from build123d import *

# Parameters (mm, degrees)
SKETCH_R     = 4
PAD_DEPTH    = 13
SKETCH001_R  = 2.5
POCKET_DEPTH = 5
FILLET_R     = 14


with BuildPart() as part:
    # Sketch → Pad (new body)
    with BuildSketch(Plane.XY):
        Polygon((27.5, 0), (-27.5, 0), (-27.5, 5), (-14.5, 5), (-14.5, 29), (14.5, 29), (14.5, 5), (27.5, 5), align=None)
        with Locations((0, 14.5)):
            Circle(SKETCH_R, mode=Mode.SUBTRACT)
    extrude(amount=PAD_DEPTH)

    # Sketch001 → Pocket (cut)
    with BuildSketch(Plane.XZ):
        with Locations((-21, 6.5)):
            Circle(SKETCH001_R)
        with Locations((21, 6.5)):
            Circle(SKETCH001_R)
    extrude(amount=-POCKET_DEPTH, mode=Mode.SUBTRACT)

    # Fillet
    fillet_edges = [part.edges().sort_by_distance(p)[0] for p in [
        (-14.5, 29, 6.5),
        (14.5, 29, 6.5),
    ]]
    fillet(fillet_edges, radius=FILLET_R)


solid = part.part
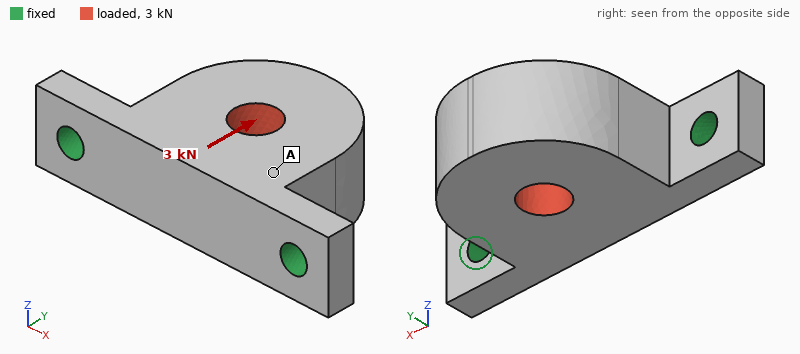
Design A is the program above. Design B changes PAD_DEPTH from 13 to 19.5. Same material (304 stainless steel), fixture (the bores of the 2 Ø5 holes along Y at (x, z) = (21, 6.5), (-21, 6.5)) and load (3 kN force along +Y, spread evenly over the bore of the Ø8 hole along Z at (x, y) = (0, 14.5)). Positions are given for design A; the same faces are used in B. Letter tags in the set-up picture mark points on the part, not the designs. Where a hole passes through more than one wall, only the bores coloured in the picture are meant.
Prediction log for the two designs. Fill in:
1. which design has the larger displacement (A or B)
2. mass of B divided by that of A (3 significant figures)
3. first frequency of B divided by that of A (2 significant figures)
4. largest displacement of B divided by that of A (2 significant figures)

B
1.51
0.94
2.5
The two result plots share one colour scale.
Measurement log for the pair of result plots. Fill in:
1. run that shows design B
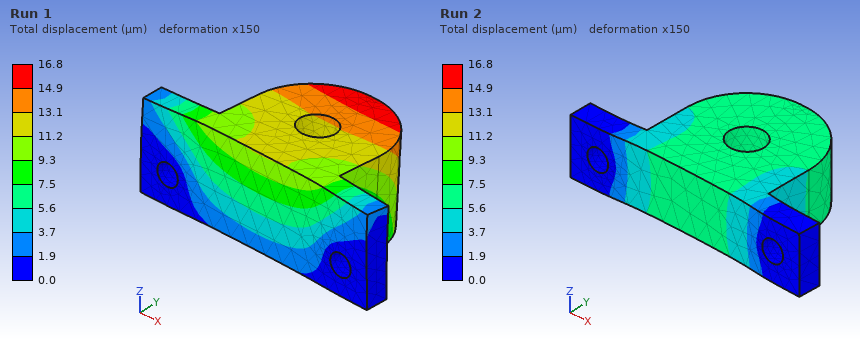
Run 1
